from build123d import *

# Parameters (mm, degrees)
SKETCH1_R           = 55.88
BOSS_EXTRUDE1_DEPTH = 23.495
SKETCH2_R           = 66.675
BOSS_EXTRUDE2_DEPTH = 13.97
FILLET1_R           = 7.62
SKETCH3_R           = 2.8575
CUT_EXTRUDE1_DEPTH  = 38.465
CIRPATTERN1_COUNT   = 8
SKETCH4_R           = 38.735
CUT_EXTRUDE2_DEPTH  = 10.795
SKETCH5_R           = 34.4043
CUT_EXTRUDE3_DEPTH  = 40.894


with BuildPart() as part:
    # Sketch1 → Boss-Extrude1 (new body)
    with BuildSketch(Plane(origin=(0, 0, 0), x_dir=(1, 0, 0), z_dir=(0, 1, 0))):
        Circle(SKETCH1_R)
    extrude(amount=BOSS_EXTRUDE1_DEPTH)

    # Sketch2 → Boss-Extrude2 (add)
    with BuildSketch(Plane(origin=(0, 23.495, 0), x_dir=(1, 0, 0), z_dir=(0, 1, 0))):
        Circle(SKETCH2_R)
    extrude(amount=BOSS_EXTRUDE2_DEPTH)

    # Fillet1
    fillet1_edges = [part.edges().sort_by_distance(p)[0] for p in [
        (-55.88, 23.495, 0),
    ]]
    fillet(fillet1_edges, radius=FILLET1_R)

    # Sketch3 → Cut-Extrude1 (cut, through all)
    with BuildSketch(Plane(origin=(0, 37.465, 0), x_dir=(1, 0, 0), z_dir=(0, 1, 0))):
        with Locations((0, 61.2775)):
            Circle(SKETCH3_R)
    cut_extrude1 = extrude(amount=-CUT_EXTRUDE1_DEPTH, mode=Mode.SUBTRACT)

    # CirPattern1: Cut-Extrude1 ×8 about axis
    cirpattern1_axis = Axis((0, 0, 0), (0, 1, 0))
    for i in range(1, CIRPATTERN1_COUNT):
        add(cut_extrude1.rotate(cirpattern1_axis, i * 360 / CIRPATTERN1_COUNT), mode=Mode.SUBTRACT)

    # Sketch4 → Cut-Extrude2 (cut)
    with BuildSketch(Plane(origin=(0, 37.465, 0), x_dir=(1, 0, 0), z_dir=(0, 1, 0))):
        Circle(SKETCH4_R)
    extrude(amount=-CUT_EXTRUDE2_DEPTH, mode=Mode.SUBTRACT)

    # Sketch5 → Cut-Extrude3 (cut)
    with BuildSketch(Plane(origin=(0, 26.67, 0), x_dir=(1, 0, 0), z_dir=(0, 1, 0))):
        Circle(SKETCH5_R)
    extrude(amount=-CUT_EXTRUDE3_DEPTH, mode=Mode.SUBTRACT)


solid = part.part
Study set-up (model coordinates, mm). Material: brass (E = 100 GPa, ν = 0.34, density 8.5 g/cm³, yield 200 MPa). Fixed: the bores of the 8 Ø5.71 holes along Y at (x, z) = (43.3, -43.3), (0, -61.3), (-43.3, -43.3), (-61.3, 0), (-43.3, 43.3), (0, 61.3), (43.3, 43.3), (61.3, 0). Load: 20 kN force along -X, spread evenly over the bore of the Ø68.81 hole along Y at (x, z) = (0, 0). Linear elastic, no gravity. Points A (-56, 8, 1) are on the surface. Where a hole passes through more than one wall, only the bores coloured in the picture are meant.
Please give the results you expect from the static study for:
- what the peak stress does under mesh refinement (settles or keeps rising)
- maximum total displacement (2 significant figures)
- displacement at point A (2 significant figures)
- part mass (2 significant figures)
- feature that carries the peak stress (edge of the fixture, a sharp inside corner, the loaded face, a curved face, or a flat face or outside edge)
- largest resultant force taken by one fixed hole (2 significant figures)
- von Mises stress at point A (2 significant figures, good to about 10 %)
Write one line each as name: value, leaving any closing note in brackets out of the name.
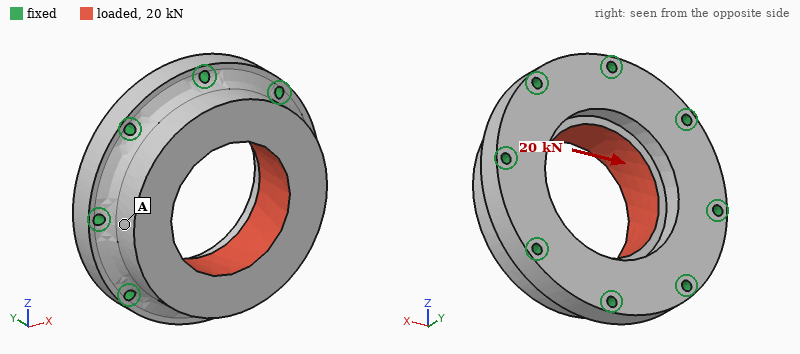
what the peak stress does under mesh refinement: keeps rising
maximum total displacement: 6.5 µm
displacement at point A: 4.1 µm
part mass: 2.4 kg
feature that carries the peak stress: edge of the fixture
largest resultant force taken by one fixed hole: 3.2 kN
von Mises stress at point A: 3.9 MPa
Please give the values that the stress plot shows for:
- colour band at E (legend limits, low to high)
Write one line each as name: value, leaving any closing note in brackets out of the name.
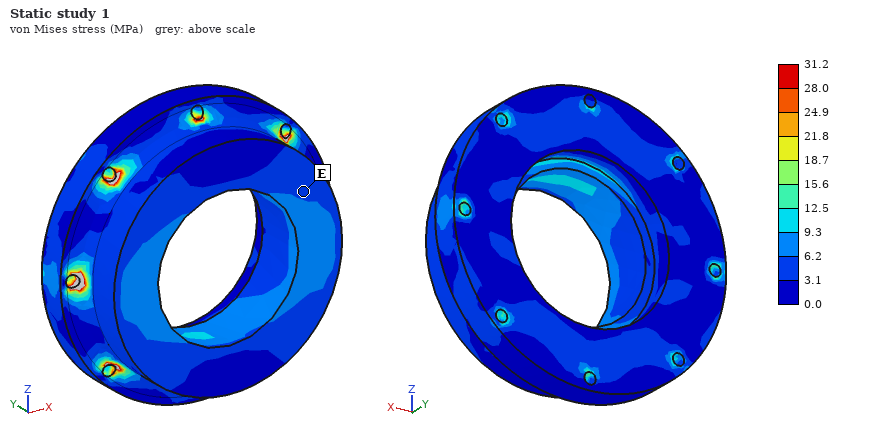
colour band at E: 3.1 to 6.2 MPa
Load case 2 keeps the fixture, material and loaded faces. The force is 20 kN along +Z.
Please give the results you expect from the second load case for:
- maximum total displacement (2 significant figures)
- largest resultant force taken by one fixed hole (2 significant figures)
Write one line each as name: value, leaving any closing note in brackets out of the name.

maximum total displacement: 6.4 µm
largest resultant force taken by one fixed hole: 3.2 kN
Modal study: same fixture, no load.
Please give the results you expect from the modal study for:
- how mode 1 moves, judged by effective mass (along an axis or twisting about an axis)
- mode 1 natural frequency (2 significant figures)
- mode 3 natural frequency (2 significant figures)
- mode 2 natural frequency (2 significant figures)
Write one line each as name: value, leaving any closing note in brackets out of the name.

how mode 1 moves, judged by effective mass: along Y
mode 1 natural frequency: 8300 Hz
mode 3 natural frequency: 9700 Hz
mode 2 natural frequency: 9700 Hz
